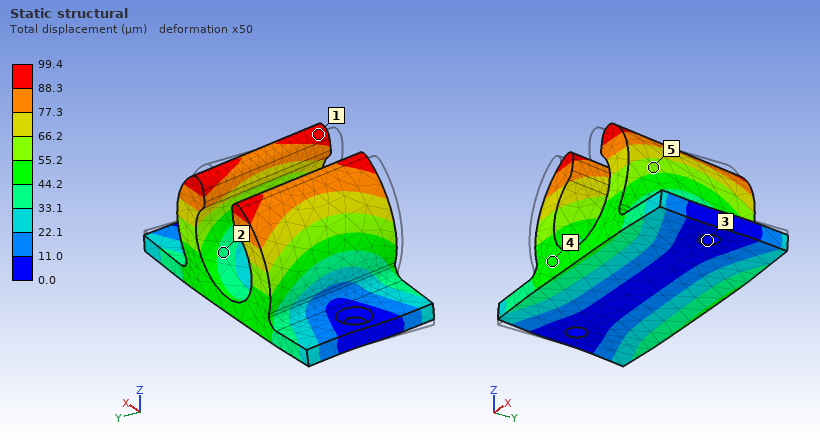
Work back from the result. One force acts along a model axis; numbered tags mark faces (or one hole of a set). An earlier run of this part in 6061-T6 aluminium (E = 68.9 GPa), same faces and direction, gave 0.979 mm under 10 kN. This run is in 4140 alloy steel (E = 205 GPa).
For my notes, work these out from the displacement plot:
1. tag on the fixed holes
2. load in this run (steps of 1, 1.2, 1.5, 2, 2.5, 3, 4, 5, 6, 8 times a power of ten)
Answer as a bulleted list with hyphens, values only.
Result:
- 3
- 3 kN
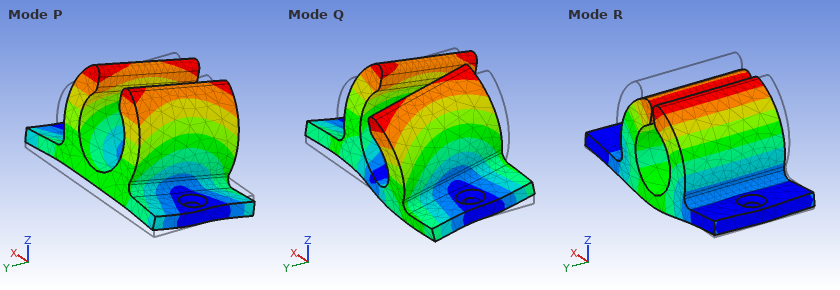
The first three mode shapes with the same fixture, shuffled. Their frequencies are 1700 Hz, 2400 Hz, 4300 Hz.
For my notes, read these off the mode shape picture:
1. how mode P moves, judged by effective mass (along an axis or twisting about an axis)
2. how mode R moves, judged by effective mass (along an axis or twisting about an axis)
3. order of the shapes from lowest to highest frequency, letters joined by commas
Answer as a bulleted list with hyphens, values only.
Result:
- along Y
- along Z
- P, R, Q
